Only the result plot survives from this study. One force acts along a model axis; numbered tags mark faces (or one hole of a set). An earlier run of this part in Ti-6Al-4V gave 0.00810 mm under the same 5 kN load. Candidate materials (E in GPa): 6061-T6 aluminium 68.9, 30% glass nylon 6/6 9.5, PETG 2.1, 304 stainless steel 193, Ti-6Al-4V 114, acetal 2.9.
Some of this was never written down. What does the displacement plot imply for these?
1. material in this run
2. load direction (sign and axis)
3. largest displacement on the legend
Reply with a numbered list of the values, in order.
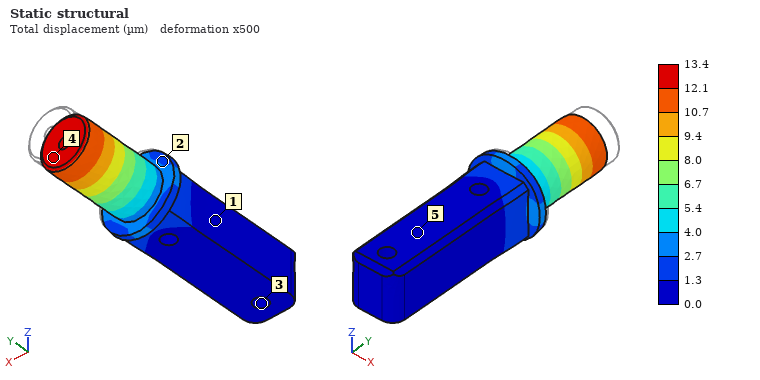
1. 6061-T6 aluminium
2. -Y
3. 13.4 µm
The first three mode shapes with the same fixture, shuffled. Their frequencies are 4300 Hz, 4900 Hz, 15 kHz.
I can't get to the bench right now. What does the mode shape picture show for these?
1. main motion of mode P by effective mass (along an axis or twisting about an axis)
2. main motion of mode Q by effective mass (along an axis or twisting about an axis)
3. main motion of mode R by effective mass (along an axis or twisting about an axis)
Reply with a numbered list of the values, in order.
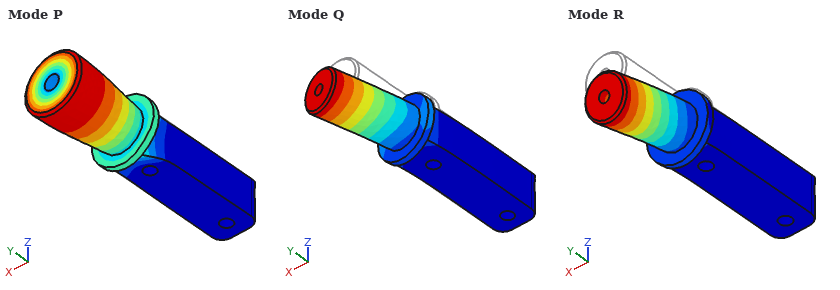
1. twisting about Y
2. along X
3. along Z
